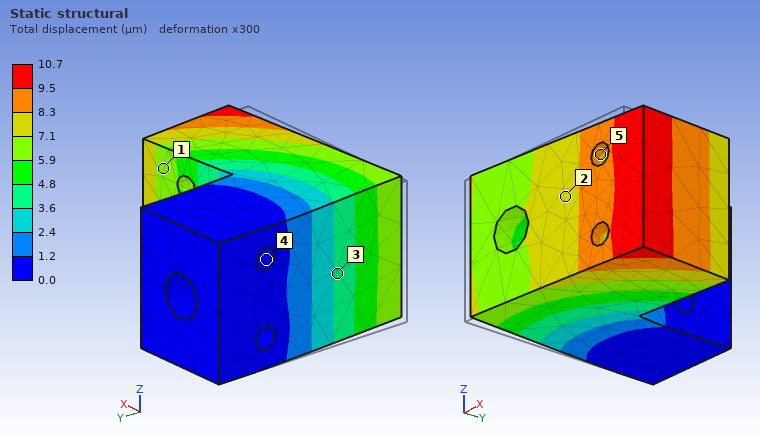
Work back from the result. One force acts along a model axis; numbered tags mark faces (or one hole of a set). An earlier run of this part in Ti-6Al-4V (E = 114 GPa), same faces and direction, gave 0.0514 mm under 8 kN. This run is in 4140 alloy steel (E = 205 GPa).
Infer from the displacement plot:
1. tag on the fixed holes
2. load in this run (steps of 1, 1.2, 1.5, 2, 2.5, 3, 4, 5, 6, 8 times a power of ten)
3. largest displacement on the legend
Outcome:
4
3 kN
10.7 µm
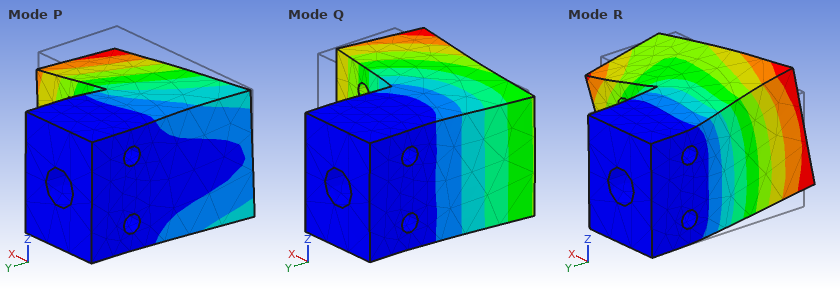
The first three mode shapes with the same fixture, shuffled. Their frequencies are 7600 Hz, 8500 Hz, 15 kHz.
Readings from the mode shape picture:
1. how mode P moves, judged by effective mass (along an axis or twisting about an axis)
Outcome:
along Z
